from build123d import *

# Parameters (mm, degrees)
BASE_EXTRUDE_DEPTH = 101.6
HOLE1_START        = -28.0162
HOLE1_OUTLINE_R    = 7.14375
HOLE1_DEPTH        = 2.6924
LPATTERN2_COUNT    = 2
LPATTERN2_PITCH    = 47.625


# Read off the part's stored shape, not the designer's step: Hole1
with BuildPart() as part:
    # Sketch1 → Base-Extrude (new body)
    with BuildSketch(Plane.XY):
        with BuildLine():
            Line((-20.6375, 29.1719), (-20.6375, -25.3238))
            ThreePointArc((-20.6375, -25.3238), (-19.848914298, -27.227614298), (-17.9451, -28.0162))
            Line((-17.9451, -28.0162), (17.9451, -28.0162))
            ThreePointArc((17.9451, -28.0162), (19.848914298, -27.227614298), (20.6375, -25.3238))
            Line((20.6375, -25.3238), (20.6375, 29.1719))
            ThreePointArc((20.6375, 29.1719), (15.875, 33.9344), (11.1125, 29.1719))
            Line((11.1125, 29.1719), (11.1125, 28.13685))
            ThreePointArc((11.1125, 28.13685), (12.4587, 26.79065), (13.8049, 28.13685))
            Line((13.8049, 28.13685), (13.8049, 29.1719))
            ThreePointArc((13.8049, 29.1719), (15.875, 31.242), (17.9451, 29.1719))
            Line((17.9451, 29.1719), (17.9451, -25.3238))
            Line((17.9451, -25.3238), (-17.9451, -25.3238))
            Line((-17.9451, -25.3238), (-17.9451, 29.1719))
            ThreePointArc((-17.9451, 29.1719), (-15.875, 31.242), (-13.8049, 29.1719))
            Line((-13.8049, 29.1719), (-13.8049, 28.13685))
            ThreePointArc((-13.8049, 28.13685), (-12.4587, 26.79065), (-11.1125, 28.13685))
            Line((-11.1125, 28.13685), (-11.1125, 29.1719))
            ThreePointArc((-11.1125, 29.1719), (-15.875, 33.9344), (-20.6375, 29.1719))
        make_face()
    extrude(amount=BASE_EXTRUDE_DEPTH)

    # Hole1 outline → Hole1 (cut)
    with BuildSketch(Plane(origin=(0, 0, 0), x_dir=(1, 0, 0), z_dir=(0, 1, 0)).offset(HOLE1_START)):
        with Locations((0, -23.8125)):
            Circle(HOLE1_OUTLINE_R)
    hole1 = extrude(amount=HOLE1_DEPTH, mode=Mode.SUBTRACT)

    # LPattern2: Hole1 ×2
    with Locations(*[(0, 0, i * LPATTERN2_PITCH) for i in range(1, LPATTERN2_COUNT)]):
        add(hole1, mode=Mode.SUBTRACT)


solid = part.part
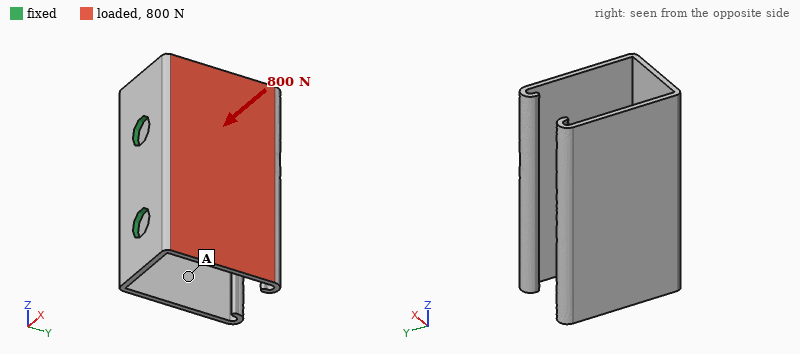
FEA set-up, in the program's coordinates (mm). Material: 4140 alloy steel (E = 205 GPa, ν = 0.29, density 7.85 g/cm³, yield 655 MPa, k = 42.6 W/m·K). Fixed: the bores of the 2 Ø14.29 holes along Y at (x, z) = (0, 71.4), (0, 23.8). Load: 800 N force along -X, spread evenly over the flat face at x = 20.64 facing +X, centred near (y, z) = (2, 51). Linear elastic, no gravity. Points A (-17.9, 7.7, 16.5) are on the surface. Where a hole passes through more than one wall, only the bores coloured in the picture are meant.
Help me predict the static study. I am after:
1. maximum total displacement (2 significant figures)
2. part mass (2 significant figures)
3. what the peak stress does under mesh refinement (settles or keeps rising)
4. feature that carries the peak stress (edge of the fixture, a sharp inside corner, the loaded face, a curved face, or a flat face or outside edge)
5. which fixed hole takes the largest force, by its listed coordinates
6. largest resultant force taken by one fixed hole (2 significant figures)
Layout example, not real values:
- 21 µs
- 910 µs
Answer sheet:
- 1.1 mm
- 370 g
- keeps rising
- edge of the fixture
- (0, 71.4)
- 430 N
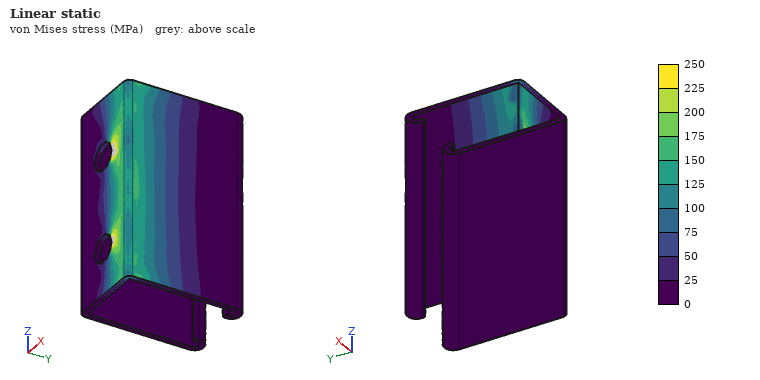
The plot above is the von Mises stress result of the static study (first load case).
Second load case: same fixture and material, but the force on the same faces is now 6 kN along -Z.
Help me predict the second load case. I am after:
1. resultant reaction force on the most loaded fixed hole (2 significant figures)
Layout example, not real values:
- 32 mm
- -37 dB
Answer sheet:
- 4.7 kN
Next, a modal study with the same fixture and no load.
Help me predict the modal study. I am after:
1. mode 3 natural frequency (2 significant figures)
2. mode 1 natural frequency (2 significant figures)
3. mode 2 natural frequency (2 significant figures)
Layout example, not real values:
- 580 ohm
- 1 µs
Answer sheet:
- 760 Hz
- 380 Hz
- 380 Hz
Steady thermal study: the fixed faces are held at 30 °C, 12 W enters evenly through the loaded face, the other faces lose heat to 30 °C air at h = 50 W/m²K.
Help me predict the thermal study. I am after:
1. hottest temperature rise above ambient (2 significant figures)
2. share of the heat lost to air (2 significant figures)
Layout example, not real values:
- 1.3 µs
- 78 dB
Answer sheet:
- 17 K
- 63 %
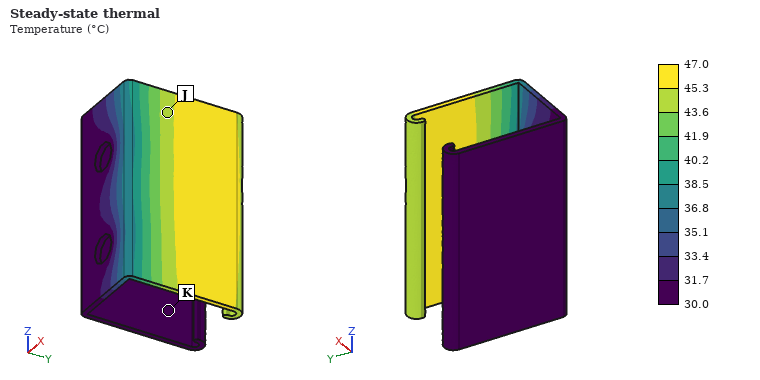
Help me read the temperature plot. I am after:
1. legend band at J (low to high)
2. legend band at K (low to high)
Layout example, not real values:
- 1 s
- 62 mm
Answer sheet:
- 43.6 to 45.3 °C
- 30.0 to 31.7 °C
